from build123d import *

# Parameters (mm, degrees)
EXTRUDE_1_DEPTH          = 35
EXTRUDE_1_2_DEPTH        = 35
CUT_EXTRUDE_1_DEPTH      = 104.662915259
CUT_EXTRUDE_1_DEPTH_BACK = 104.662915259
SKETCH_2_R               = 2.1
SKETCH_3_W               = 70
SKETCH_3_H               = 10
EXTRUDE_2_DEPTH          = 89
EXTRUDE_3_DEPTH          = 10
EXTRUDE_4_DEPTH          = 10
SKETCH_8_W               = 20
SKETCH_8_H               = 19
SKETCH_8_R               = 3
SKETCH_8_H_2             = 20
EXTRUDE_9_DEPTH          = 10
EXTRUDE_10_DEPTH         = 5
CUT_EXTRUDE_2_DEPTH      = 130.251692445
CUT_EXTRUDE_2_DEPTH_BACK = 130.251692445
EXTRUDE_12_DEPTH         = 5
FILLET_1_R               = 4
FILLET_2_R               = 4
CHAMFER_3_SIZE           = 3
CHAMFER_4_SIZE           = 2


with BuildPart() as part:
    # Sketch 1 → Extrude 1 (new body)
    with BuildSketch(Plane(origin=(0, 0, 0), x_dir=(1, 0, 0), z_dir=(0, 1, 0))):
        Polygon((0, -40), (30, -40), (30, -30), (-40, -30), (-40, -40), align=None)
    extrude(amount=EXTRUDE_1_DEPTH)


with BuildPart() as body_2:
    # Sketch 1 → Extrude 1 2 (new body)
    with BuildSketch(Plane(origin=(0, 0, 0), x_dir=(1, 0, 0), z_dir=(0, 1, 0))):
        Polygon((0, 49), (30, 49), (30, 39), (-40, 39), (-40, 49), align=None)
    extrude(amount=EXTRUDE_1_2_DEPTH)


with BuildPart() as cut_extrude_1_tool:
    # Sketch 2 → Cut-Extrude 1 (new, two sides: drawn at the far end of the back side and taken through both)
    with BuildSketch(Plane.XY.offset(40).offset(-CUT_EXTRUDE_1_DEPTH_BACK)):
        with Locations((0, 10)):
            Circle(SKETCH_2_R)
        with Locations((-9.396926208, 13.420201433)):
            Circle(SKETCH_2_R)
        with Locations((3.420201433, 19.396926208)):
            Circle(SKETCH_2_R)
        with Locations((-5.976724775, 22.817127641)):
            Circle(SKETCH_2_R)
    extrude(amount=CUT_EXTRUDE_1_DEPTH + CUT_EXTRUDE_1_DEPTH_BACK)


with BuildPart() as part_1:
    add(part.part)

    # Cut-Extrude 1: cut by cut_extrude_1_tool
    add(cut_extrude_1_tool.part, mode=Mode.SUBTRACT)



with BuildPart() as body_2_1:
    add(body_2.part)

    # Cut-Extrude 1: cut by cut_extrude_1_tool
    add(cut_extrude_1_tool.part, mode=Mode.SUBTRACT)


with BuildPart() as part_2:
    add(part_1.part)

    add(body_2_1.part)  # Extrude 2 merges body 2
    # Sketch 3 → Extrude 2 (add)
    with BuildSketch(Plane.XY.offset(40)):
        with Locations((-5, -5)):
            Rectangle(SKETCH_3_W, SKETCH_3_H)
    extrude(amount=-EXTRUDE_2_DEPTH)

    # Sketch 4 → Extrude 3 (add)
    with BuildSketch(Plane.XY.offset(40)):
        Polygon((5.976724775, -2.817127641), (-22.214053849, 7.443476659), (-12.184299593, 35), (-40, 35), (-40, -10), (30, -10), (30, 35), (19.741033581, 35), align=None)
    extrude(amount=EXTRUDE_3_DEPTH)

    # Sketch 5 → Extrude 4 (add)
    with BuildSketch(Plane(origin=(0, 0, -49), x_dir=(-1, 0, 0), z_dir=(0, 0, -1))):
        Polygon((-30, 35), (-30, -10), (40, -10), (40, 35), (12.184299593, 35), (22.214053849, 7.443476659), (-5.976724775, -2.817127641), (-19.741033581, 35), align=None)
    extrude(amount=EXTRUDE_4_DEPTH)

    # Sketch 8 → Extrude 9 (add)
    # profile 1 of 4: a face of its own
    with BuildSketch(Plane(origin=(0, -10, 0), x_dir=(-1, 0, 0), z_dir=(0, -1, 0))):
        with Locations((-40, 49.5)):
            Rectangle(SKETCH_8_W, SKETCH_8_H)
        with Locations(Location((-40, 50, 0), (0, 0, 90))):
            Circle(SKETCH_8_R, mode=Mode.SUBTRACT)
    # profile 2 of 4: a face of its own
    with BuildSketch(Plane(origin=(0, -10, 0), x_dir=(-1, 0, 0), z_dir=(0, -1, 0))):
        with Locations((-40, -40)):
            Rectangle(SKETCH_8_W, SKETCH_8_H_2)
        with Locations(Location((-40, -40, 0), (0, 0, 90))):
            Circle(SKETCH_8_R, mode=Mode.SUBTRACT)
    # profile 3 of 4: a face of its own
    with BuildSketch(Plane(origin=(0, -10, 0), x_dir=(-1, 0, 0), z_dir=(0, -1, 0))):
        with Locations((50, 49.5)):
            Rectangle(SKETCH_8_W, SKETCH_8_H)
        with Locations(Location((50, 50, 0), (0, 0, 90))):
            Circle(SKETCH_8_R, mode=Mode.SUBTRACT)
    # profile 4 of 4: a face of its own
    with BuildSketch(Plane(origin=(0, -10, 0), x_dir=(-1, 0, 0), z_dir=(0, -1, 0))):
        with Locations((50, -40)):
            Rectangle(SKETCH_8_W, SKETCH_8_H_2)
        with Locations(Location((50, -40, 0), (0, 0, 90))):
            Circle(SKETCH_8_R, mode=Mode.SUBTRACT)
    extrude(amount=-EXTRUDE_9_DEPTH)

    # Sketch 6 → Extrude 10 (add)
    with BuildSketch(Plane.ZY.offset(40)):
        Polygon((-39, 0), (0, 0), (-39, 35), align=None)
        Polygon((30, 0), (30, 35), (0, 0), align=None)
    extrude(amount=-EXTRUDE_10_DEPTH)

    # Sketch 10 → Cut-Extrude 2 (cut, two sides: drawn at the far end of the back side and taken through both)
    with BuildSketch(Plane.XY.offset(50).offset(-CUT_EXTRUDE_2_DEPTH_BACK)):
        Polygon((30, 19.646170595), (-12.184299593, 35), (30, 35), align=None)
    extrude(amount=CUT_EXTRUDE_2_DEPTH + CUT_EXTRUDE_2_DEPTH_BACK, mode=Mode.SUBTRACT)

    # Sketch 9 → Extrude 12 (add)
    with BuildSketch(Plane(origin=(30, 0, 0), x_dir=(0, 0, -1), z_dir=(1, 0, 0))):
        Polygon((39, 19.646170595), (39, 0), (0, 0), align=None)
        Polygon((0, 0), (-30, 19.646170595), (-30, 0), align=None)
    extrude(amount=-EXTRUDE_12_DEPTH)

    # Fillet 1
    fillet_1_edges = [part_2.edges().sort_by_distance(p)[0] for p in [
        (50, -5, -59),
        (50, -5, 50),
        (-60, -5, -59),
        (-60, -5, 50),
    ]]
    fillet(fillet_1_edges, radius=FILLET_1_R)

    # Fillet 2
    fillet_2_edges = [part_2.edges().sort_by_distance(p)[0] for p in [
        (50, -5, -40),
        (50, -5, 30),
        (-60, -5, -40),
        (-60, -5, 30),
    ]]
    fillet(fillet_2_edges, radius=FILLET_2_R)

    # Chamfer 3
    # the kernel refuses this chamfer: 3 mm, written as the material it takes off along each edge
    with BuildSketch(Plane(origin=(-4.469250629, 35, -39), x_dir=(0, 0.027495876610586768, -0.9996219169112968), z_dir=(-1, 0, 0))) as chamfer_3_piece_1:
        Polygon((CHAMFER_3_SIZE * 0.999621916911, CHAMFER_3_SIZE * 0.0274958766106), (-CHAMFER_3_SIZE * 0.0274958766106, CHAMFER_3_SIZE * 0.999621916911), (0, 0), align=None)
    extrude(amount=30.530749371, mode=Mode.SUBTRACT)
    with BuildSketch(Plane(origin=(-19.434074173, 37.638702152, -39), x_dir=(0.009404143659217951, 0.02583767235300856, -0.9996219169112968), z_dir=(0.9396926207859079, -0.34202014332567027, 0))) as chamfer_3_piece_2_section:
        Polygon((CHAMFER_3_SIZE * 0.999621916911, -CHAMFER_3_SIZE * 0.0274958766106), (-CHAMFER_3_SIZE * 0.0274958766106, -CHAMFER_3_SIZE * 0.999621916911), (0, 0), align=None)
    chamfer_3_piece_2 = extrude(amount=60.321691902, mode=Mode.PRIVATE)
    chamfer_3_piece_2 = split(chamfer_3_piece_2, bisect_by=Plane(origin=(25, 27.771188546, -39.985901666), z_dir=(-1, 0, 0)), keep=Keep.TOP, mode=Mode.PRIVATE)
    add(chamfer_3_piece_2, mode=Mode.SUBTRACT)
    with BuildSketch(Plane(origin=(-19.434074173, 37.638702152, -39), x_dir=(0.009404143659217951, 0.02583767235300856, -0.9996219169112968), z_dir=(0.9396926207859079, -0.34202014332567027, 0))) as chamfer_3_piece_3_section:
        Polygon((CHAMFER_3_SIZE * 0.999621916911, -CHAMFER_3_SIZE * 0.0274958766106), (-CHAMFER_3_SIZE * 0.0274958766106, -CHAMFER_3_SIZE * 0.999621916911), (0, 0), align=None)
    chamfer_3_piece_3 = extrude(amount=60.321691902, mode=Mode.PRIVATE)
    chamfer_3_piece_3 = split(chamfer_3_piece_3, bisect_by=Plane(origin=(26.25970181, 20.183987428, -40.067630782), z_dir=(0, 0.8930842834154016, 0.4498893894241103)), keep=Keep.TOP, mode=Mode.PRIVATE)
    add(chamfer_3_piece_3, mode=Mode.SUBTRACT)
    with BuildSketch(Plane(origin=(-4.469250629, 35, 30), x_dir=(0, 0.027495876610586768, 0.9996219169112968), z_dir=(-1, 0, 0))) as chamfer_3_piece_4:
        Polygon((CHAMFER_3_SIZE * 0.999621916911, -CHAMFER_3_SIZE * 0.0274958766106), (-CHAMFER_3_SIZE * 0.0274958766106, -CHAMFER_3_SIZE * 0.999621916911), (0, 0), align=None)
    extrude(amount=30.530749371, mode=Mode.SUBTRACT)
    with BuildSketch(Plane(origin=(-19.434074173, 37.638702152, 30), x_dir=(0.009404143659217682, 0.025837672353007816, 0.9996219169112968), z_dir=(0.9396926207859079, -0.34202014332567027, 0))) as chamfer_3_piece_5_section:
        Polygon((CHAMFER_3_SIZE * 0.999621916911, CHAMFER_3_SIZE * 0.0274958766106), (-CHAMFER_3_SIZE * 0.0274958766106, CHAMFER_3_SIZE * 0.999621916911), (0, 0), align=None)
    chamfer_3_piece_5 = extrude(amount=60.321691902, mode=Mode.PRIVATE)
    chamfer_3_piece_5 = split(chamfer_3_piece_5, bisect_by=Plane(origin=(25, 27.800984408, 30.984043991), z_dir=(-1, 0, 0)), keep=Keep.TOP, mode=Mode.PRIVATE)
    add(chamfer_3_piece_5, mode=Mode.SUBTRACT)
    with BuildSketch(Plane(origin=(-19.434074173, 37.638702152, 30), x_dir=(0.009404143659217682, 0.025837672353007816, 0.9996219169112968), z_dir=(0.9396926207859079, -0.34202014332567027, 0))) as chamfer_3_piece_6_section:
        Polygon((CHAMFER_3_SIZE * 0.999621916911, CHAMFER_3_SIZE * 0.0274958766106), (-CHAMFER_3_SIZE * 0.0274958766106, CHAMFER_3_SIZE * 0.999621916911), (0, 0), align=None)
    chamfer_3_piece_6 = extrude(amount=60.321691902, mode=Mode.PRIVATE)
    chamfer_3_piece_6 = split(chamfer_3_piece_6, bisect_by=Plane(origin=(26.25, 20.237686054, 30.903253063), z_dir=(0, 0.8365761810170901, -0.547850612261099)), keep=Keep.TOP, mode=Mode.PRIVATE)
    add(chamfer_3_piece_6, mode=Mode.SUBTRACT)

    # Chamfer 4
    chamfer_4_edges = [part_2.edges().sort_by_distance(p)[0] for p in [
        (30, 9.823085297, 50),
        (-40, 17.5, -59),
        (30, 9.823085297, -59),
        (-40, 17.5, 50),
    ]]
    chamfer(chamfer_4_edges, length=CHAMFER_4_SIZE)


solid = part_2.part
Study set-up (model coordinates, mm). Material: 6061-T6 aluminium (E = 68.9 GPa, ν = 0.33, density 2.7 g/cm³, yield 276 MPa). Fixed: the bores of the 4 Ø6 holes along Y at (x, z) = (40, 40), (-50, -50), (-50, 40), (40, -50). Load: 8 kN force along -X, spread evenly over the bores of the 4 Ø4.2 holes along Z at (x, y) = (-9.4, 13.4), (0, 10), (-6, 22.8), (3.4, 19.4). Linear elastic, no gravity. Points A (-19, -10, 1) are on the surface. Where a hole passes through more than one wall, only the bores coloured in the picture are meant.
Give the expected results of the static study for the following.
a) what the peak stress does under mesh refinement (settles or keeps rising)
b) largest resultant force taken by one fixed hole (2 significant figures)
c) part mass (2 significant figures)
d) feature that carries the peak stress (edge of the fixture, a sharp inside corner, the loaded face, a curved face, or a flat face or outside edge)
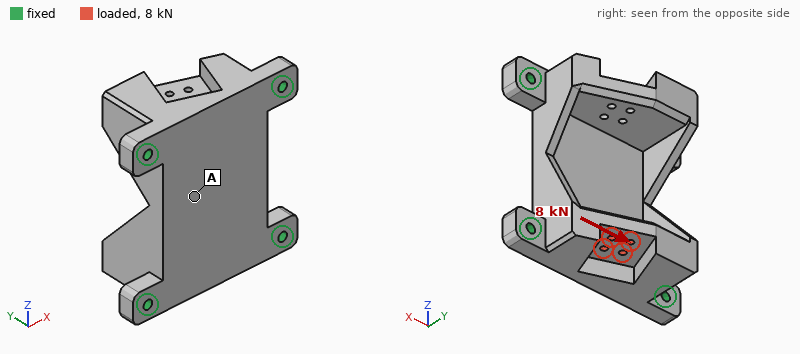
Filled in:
keeps rising
4.3 kN
450 g
edge of the fixture
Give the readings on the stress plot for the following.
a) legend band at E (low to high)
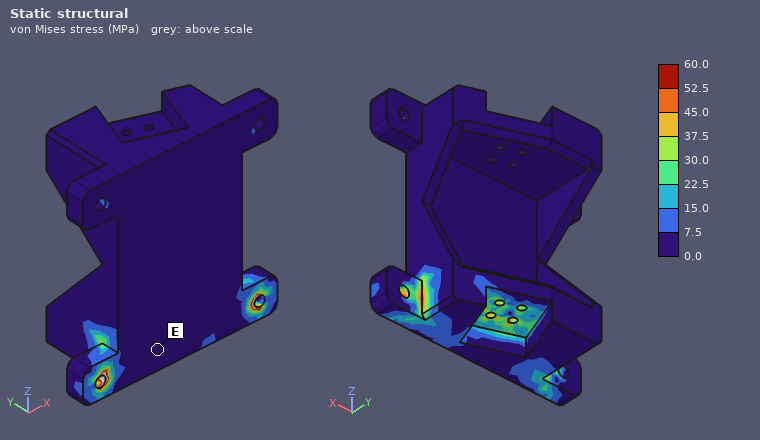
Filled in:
0.0 to 7.5 MPa
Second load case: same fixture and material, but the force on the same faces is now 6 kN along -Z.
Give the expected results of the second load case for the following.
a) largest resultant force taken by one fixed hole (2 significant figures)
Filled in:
2.0 kN
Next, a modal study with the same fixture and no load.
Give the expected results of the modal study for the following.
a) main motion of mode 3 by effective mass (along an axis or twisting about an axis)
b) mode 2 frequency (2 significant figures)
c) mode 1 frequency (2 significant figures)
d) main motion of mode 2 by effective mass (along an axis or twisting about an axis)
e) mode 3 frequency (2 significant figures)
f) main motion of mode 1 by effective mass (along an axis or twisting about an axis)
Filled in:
along Y
5300 Hz
3100 Hz
along Z
6200 Hz
along Y
